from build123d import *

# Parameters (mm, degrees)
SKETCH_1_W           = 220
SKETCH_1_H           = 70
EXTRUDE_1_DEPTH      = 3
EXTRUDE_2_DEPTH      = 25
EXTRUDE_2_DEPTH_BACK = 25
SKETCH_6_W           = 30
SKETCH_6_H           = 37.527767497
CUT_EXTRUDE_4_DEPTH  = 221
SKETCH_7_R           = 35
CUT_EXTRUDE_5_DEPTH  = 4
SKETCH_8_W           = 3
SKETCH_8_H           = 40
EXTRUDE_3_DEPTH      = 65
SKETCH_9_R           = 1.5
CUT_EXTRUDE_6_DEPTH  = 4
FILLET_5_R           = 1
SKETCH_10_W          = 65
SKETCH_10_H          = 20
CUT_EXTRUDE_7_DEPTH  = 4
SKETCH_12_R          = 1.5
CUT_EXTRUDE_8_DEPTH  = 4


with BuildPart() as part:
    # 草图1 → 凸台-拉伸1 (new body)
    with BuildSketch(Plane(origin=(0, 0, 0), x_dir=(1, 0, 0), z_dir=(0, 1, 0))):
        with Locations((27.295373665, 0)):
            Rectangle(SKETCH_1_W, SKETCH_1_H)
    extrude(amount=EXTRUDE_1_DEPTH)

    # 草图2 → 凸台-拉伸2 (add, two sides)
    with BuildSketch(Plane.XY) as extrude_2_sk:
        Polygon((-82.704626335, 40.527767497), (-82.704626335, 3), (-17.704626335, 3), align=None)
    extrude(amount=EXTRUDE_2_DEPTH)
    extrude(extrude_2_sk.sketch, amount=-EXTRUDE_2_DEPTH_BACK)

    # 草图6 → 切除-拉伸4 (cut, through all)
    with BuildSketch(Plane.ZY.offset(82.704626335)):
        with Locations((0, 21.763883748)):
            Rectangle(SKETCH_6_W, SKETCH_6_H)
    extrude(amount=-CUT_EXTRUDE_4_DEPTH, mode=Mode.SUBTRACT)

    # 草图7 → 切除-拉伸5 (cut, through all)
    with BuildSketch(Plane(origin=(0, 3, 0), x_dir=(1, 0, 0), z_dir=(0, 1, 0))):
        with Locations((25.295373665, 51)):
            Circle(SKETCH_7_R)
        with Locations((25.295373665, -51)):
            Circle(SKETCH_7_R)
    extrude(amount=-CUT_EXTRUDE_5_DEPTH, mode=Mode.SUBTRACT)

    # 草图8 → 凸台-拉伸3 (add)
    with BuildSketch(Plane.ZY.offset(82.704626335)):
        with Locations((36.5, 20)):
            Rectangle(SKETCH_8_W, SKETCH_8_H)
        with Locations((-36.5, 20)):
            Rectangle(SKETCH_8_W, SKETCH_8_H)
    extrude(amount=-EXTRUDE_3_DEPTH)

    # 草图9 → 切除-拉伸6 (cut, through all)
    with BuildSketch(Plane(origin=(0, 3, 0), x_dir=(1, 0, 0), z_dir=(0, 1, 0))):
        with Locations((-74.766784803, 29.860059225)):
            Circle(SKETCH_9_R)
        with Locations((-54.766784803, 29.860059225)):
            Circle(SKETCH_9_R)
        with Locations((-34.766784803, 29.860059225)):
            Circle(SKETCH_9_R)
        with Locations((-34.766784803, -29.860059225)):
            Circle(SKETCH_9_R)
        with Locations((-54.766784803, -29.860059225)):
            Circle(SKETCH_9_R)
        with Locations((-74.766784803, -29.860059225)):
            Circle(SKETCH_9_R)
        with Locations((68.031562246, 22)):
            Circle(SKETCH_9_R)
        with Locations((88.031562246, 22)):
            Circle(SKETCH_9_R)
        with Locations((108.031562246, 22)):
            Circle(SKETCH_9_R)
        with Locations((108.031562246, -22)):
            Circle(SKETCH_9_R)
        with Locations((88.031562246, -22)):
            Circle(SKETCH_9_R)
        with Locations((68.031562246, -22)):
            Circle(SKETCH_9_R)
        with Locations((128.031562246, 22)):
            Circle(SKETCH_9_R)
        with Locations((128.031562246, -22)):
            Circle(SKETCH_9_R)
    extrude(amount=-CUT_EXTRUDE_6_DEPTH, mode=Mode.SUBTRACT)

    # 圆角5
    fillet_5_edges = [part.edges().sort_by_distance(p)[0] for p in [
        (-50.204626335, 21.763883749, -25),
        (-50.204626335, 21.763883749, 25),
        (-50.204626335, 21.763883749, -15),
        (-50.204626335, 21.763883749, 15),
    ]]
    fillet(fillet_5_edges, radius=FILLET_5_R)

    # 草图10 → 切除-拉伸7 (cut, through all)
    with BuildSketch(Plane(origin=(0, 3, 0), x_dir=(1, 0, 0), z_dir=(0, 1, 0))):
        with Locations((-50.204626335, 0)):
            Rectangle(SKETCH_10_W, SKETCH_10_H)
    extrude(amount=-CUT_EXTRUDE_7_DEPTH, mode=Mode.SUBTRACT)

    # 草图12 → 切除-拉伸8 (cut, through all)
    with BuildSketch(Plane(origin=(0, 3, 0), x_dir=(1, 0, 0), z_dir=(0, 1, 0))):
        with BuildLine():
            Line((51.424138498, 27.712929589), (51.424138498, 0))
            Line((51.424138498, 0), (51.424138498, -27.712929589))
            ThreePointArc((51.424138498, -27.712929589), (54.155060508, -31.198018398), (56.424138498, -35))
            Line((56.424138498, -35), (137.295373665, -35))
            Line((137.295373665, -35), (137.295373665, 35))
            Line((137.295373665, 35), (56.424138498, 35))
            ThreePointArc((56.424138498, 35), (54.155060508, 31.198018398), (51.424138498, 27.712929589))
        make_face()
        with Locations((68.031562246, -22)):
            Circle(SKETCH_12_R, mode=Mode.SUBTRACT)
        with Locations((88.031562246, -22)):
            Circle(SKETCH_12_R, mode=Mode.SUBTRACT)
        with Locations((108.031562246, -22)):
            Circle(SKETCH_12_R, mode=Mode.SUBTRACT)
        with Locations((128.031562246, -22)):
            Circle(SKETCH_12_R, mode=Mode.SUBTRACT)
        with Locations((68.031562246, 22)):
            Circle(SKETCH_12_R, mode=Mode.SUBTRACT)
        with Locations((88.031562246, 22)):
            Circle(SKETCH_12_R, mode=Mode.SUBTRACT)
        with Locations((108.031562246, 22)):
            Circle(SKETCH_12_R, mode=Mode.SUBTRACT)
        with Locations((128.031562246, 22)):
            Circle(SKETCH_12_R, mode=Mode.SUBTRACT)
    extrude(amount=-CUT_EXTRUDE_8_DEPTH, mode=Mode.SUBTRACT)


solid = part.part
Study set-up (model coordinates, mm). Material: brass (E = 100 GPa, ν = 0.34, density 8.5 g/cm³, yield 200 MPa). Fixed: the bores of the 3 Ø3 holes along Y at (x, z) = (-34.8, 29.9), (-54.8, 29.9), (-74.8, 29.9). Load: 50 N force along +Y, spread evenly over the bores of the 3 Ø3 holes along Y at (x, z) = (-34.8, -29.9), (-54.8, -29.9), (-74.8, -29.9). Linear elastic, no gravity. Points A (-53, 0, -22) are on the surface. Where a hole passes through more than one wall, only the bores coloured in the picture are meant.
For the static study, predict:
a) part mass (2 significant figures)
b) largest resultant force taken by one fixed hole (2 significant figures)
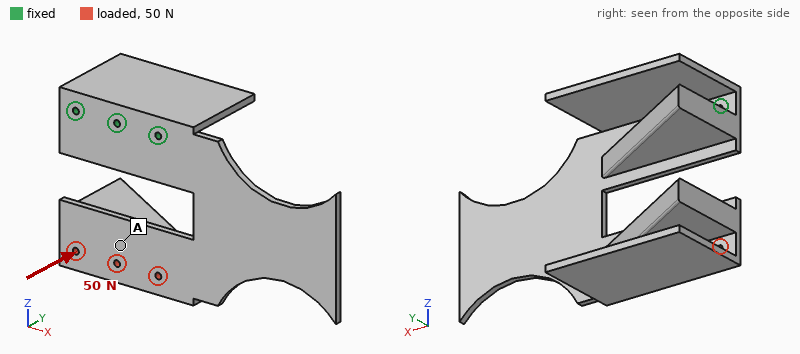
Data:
500 g
43 N
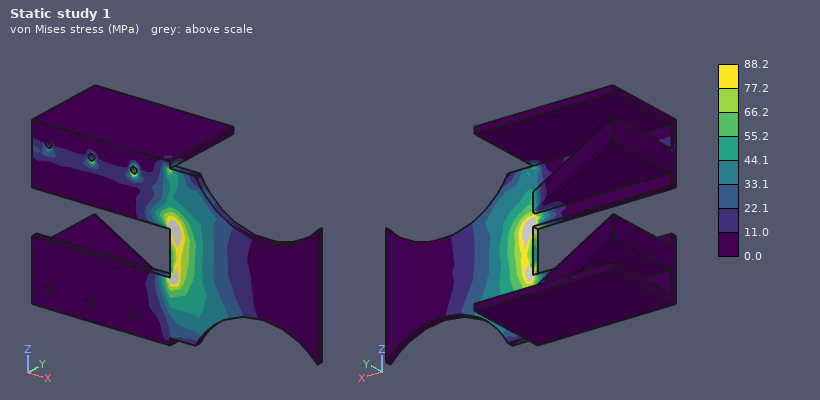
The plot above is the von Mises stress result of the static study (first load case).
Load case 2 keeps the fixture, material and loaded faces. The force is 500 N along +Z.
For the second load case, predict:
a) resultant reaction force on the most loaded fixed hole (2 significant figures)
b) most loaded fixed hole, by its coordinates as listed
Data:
260 N
(-34.8, 29.9)
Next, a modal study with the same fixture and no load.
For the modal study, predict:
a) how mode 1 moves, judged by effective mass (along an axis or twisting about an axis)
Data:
along Y
